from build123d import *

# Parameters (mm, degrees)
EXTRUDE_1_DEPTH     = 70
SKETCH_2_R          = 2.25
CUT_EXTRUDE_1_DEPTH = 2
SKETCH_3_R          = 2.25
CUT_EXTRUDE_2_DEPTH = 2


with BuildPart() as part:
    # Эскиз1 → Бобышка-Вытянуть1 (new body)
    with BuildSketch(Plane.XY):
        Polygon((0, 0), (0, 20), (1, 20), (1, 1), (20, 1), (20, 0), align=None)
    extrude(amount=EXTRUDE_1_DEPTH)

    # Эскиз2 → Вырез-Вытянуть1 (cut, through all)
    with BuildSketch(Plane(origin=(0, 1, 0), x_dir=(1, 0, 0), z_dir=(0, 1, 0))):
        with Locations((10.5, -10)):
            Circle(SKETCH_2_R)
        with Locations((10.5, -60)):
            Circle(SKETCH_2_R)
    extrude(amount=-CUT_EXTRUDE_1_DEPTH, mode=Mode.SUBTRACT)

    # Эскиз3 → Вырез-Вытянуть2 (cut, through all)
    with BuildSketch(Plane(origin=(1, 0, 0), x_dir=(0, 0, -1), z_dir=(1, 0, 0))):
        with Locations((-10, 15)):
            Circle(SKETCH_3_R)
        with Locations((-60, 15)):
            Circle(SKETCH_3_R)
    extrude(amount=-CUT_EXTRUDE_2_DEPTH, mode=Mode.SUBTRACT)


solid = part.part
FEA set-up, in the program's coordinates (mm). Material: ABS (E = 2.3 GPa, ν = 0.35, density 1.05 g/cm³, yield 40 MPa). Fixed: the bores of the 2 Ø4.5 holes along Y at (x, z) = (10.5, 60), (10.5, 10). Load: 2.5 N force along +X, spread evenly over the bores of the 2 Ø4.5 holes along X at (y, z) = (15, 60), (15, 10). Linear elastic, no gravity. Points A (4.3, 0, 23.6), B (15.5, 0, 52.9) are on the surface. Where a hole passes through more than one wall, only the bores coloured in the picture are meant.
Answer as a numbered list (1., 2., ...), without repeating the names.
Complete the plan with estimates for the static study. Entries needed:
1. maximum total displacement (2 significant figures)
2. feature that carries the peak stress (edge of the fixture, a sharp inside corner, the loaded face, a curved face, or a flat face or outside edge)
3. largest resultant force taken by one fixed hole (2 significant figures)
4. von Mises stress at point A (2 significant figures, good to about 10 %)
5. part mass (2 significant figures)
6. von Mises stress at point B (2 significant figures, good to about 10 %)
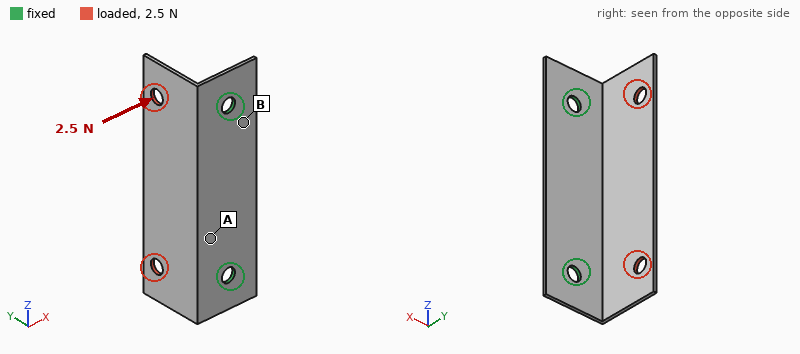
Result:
1. 0.90 mm
2. a flat face or outside edge
3. 1.3 N
4. 1.9 MPa
5. 2.8 g
6. 0.75 MPa
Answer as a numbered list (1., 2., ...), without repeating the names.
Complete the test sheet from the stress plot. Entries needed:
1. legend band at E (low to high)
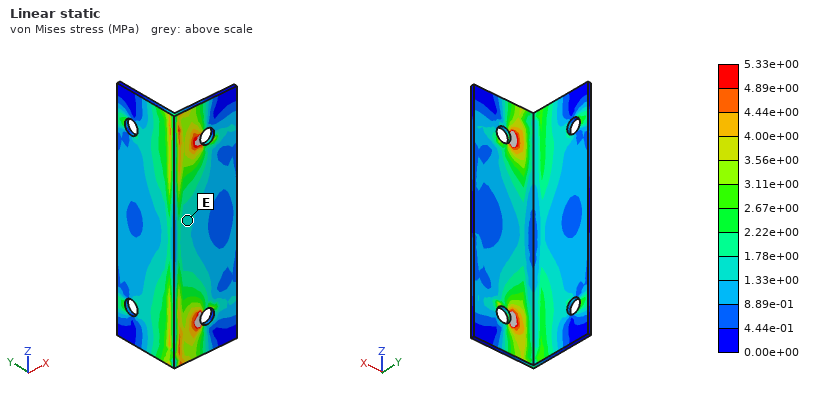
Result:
1. 1.33e+00 to 1.78e+00 MPa
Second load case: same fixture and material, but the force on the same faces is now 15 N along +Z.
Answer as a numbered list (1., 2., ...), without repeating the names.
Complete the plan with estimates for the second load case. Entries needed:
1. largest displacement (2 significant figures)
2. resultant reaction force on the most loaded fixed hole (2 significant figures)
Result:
1. 0.58 mm
2. 9.0 N
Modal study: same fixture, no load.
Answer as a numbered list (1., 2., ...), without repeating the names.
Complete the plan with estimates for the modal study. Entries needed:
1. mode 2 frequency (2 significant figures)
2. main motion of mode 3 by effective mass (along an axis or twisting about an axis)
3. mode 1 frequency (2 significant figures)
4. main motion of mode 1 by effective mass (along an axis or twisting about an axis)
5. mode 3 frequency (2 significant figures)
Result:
1. 520 Hz
2. along Y
3. 350 Hz
4. along X
5. 800 Hz
